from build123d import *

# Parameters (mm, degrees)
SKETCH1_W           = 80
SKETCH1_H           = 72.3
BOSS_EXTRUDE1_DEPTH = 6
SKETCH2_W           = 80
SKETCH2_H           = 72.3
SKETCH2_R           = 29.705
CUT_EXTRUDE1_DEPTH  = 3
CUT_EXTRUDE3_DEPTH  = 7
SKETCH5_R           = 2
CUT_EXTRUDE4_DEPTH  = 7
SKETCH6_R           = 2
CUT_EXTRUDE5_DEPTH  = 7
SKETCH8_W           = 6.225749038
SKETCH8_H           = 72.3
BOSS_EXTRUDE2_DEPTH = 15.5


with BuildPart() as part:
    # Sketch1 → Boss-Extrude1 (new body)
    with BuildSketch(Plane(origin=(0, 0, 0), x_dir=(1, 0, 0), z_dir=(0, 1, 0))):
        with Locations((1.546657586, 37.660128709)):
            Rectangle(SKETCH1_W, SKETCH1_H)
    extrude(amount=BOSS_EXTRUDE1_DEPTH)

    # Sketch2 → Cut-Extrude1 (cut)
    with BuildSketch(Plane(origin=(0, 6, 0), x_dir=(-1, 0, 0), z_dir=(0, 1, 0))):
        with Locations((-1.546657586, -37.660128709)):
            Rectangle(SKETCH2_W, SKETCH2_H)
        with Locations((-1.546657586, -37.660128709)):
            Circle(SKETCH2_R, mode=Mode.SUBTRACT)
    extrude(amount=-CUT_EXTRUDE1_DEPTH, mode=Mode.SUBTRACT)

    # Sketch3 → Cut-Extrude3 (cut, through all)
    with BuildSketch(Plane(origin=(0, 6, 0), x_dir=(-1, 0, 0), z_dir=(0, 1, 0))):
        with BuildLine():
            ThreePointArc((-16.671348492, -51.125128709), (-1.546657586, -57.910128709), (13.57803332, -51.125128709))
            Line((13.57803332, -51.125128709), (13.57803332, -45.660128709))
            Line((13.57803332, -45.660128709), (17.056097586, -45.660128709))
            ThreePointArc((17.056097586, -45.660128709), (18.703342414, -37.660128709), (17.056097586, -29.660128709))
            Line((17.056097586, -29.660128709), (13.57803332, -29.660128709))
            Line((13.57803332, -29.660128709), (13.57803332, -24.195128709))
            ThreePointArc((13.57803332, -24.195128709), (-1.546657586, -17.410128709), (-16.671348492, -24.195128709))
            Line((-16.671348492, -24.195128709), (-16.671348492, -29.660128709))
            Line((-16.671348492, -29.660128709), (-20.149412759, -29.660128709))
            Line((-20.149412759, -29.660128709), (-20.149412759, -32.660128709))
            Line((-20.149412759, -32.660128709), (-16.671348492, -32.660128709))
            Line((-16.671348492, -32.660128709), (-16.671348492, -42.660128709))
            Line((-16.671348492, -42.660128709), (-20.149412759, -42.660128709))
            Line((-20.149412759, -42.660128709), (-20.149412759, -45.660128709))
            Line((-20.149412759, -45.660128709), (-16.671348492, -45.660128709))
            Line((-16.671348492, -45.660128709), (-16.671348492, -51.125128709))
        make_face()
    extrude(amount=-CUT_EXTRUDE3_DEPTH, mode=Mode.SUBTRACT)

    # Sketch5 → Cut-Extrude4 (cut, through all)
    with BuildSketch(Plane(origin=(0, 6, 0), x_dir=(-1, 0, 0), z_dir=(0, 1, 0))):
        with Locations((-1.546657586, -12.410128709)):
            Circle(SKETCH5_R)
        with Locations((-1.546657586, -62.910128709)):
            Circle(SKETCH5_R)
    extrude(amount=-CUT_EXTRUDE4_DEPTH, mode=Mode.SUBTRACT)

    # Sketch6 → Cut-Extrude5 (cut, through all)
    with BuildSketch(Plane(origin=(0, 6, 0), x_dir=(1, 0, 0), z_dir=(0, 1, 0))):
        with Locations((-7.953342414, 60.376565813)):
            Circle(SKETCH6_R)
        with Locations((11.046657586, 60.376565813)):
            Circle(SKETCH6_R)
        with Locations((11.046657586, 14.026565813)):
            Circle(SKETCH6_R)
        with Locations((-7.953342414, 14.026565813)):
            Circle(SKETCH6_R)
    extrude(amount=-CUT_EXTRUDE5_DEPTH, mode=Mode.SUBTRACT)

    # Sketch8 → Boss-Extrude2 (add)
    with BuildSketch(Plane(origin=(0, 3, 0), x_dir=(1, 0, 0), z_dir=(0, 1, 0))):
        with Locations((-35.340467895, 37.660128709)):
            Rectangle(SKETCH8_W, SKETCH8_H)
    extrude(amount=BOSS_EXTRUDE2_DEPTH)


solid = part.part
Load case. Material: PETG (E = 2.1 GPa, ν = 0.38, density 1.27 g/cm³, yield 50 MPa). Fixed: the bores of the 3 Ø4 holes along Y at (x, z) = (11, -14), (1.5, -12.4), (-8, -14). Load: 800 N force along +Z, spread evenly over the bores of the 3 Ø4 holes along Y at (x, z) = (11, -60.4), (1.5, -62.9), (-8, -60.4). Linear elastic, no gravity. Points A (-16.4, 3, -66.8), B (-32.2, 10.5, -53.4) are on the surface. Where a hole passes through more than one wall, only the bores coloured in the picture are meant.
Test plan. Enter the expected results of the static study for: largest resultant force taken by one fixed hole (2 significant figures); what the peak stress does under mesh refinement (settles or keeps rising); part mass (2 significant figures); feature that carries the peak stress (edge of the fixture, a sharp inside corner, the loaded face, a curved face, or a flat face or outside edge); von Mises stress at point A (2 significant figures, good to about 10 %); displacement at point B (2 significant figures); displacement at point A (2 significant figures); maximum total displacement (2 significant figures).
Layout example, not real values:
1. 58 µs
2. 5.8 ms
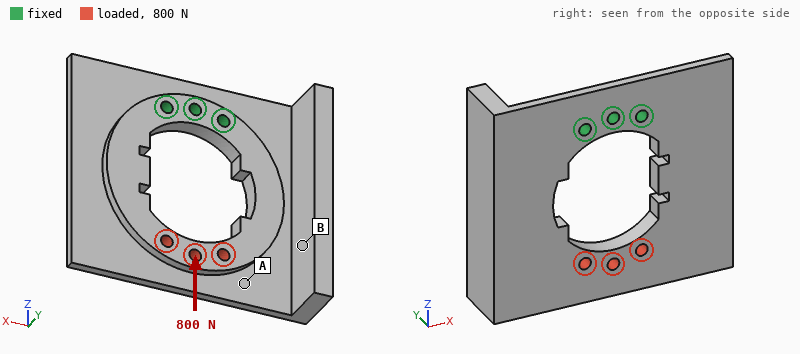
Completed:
1. 500 N
2. keeps rising
3. 32 g
4. edge of the fixture
5. 6.6 MPa
6. 0.38 mm
7. 0.46 mm
8. 0.67 mm
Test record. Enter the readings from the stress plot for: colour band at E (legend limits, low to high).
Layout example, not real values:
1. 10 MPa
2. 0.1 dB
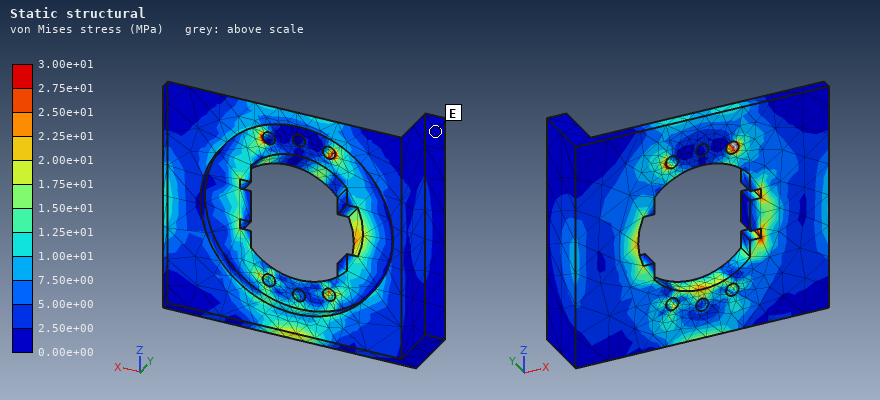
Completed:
1. 0.00e+00 to 2.50e+00 MPa
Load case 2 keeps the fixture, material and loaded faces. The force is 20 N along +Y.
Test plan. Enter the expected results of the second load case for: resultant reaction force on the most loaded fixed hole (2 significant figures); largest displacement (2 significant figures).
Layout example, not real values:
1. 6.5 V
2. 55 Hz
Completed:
1. 19 N
2. 1.2 mm
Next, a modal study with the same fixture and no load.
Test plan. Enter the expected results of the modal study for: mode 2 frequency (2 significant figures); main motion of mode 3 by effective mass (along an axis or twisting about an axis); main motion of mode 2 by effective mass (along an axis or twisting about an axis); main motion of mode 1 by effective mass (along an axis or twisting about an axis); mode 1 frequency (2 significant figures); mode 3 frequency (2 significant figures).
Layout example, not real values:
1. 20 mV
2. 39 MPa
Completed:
1. 300 Hz
2. along X
3. twisting about Z
4. along Y
5. 200 Hz
6. 500 Hz
